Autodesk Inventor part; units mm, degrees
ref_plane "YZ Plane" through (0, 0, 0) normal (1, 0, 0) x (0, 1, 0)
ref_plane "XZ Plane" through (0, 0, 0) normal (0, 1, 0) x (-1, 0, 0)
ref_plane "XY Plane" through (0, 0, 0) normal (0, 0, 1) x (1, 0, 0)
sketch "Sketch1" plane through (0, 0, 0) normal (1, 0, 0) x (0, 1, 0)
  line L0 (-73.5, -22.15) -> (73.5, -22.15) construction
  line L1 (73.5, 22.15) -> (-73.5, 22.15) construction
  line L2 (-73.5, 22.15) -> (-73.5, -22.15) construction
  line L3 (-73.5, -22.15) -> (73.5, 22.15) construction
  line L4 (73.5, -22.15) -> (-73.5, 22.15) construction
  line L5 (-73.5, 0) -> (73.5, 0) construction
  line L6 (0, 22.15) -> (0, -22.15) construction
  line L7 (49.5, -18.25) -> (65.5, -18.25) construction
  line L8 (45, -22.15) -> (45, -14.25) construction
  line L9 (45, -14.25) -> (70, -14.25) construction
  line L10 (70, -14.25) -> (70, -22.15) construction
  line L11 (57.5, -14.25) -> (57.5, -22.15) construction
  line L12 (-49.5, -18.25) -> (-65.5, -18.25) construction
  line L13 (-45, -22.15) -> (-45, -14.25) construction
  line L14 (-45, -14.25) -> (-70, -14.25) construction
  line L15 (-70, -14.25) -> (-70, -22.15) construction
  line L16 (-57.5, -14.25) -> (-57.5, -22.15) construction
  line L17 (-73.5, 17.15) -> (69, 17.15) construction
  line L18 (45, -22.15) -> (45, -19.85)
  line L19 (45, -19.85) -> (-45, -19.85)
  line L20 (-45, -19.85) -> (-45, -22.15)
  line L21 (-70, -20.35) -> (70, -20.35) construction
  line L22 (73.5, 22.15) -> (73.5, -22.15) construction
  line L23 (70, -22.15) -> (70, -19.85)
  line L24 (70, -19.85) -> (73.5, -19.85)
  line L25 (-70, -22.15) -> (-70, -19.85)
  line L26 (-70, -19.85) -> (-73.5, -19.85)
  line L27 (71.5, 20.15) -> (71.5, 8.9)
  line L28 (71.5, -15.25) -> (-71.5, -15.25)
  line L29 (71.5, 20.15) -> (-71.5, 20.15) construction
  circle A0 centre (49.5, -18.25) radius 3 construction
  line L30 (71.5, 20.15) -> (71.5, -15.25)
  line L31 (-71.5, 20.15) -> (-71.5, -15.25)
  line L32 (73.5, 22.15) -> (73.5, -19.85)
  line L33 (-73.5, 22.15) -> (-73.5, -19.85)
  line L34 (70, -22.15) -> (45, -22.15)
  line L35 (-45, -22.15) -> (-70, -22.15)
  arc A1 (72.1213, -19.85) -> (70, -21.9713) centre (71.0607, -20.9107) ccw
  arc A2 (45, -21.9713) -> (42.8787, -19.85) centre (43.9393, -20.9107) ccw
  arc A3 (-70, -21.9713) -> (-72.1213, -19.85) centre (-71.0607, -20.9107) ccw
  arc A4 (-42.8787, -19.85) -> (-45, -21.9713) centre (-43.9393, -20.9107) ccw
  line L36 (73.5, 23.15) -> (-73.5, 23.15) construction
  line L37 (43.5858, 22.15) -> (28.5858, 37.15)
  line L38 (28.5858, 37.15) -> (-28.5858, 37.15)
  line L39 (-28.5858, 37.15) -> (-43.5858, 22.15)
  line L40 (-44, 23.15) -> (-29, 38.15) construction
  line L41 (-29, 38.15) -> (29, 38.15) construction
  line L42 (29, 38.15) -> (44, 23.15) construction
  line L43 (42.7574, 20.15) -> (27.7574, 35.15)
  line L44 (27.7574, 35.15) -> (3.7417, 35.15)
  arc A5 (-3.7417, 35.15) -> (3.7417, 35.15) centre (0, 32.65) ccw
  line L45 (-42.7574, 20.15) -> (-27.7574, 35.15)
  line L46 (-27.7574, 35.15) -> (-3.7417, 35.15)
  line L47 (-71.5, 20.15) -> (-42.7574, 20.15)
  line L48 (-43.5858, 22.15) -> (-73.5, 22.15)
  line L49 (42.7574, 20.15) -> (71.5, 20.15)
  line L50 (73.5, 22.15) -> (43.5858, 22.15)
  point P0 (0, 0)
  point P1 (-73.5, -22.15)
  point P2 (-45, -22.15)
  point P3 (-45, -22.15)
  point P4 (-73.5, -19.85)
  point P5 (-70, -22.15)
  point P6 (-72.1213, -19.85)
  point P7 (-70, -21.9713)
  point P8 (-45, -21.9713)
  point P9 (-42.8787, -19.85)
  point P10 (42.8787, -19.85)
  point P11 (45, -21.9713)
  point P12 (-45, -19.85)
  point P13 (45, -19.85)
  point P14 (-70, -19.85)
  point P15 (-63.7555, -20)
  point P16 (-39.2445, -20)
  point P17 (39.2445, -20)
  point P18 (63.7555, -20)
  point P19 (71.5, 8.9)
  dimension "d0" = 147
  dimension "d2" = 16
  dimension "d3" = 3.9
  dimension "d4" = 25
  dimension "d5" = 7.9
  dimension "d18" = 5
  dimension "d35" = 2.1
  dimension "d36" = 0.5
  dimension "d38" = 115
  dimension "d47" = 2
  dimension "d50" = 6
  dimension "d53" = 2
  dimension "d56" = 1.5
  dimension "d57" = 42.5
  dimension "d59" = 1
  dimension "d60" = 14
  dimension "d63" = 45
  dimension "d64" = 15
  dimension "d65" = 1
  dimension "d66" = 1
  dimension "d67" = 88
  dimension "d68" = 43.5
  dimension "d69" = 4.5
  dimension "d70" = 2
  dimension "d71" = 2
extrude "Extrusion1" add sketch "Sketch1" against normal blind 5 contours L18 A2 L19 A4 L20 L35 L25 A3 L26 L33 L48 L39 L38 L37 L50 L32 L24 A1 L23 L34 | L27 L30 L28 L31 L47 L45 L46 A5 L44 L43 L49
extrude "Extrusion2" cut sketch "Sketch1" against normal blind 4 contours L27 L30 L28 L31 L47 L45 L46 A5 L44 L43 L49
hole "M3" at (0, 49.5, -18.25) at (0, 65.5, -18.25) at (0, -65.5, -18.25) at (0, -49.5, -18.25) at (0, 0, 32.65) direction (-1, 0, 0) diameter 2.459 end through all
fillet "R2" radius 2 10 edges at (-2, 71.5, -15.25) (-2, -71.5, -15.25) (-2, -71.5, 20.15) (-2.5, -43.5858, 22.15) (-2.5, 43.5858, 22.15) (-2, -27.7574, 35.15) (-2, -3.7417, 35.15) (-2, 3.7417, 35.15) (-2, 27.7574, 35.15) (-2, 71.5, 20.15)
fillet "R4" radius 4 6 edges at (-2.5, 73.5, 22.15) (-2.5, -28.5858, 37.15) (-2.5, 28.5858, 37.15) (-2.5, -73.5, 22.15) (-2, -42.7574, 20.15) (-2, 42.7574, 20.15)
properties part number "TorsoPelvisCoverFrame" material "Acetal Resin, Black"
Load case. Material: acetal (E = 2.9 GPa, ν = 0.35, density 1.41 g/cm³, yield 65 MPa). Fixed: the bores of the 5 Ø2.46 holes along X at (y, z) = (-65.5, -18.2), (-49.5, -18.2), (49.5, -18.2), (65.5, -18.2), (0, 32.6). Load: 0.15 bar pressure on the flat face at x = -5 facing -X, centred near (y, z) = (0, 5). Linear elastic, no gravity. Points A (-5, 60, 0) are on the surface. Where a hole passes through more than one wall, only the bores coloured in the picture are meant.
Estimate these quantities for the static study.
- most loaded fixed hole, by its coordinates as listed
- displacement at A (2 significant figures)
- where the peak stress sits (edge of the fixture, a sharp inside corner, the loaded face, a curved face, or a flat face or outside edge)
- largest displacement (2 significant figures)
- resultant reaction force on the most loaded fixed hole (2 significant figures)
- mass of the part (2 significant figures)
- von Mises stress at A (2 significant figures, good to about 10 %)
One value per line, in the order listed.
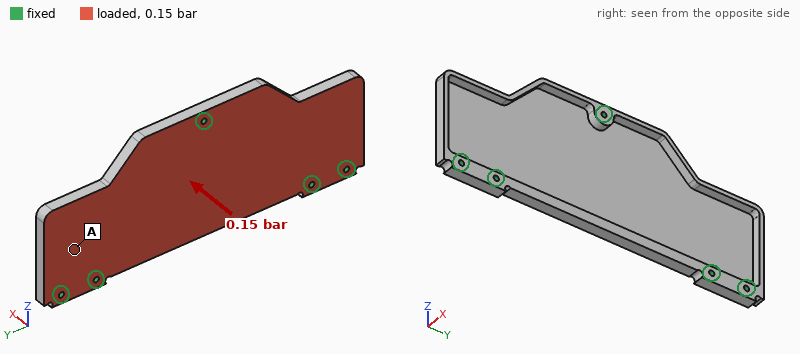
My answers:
(0, 32.6)
0.61 mm
the loaded face
1.4 mm
57 N
18 g
2.8 MPa
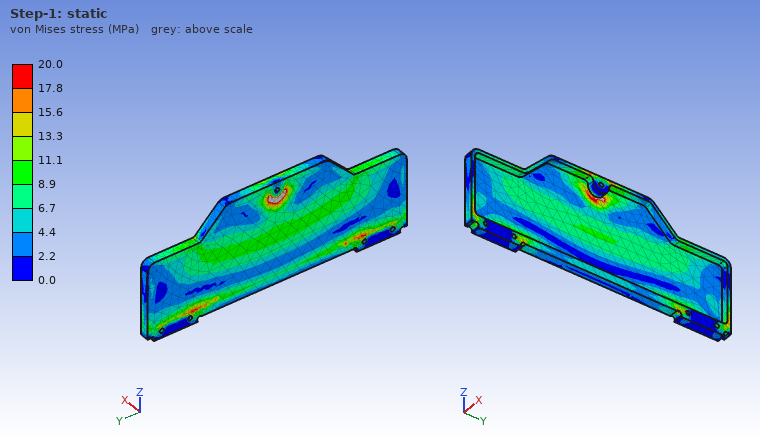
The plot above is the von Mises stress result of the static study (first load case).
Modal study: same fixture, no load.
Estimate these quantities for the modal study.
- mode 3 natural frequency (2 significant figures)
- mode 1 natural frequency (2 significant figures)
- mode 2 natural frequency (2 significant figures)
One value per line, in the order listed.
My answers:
570 Hz
450 Hz
450 Hz
